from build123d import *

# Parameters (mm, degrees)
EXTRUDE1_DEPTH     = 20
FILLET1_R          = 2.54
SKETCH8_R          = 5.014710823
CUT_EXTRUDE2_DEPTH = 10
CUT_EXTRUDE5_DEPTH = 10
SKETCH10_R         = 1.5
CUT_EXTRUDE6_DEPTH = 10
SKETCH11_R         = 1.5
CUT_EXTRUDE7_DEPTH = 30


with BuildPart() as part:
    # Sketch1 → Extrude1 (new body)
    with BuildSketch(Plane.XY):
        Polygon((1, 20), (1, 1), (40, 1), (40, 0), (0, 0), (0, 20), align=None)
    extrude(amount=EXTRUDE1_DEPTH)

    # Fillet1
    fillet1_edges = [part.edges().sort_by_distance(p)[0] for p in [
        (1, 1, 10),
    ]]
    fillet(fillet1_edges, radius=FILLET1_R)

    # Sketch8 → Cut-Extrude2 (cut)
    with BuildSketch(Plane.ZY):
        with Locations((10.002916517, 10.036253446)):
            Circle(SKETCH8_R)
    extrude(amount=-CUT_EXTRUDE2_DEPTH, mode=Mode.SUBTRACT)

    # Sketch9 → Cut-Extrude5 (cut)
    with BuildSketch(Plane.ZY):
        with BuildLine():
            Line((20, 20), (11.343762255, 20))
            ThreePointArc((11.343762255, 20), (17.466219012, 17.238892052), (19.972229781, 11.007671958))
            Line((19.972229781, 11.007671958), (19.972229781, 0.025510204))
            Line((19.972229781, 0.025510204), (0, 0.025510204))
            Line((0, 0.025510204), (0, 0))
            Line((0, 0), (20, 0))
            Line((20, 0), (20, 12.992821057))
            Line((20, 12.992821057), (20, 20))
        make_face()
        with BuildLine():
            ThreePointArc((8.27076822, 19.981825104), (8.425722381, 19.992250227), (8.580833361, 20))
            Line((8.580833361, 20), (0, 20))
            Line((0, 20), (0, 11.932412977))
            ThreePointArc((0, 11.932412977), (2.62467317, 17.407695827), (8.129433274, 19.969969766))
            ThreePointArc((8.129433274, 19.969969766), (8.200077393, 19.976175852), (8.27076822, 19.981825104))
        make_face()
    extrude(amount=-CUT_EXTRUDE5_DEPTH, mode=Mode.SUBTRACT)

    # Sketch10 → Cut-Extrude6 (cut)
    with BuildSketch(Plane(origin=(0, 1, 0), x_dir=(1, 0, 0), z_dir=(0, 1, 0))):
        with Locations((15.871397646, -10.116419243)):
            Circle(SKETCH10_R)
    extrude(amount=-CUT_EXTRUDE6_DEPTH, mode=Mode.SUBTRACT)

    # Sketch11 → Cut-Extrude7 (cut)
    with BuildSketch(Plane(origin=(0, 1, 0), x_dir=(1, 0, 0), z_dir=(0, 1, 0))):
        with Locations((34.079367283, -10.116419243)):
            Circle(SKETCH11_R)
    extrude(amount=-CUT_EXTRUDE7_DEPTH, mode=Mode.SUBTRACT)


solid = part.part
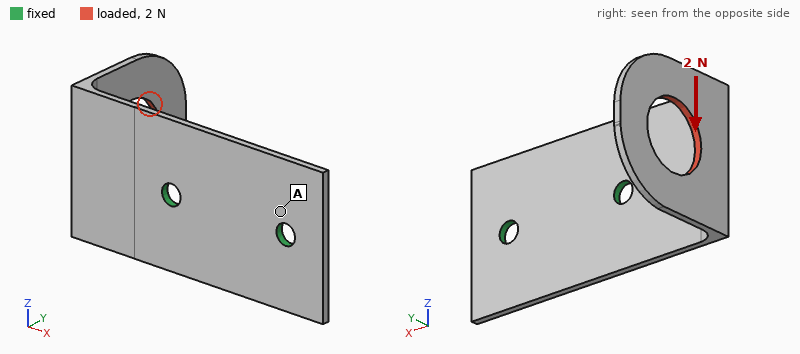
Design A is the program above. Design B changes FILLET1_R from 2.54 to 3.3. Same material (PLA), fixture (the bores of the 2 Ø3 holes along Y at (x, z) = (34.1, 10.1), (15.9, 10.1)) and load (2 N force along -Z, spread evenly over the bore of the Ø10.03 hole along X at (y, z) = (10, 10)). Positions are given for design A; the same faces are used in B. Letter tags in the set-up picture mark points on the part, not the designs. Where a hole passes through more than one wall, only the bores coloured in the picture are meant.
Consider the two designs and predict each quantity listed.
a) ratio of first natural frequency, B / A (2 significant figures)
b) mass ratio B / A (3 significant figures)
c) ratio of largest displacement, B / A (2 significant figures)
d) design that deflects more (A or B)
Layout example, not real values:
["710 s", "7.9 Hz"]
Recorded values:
["1.0", "1.02", "0.92", "A"]
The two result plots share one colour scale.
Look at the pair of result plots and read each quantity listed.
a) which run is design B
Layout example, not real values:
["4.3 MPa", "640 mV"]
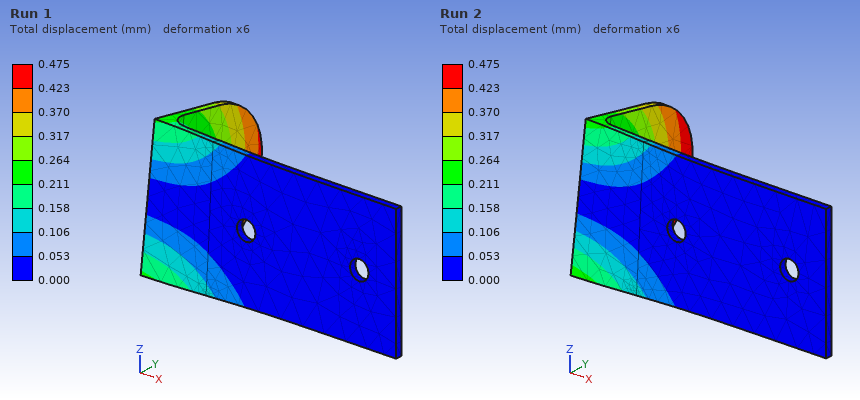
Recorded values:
["Run 1"]
